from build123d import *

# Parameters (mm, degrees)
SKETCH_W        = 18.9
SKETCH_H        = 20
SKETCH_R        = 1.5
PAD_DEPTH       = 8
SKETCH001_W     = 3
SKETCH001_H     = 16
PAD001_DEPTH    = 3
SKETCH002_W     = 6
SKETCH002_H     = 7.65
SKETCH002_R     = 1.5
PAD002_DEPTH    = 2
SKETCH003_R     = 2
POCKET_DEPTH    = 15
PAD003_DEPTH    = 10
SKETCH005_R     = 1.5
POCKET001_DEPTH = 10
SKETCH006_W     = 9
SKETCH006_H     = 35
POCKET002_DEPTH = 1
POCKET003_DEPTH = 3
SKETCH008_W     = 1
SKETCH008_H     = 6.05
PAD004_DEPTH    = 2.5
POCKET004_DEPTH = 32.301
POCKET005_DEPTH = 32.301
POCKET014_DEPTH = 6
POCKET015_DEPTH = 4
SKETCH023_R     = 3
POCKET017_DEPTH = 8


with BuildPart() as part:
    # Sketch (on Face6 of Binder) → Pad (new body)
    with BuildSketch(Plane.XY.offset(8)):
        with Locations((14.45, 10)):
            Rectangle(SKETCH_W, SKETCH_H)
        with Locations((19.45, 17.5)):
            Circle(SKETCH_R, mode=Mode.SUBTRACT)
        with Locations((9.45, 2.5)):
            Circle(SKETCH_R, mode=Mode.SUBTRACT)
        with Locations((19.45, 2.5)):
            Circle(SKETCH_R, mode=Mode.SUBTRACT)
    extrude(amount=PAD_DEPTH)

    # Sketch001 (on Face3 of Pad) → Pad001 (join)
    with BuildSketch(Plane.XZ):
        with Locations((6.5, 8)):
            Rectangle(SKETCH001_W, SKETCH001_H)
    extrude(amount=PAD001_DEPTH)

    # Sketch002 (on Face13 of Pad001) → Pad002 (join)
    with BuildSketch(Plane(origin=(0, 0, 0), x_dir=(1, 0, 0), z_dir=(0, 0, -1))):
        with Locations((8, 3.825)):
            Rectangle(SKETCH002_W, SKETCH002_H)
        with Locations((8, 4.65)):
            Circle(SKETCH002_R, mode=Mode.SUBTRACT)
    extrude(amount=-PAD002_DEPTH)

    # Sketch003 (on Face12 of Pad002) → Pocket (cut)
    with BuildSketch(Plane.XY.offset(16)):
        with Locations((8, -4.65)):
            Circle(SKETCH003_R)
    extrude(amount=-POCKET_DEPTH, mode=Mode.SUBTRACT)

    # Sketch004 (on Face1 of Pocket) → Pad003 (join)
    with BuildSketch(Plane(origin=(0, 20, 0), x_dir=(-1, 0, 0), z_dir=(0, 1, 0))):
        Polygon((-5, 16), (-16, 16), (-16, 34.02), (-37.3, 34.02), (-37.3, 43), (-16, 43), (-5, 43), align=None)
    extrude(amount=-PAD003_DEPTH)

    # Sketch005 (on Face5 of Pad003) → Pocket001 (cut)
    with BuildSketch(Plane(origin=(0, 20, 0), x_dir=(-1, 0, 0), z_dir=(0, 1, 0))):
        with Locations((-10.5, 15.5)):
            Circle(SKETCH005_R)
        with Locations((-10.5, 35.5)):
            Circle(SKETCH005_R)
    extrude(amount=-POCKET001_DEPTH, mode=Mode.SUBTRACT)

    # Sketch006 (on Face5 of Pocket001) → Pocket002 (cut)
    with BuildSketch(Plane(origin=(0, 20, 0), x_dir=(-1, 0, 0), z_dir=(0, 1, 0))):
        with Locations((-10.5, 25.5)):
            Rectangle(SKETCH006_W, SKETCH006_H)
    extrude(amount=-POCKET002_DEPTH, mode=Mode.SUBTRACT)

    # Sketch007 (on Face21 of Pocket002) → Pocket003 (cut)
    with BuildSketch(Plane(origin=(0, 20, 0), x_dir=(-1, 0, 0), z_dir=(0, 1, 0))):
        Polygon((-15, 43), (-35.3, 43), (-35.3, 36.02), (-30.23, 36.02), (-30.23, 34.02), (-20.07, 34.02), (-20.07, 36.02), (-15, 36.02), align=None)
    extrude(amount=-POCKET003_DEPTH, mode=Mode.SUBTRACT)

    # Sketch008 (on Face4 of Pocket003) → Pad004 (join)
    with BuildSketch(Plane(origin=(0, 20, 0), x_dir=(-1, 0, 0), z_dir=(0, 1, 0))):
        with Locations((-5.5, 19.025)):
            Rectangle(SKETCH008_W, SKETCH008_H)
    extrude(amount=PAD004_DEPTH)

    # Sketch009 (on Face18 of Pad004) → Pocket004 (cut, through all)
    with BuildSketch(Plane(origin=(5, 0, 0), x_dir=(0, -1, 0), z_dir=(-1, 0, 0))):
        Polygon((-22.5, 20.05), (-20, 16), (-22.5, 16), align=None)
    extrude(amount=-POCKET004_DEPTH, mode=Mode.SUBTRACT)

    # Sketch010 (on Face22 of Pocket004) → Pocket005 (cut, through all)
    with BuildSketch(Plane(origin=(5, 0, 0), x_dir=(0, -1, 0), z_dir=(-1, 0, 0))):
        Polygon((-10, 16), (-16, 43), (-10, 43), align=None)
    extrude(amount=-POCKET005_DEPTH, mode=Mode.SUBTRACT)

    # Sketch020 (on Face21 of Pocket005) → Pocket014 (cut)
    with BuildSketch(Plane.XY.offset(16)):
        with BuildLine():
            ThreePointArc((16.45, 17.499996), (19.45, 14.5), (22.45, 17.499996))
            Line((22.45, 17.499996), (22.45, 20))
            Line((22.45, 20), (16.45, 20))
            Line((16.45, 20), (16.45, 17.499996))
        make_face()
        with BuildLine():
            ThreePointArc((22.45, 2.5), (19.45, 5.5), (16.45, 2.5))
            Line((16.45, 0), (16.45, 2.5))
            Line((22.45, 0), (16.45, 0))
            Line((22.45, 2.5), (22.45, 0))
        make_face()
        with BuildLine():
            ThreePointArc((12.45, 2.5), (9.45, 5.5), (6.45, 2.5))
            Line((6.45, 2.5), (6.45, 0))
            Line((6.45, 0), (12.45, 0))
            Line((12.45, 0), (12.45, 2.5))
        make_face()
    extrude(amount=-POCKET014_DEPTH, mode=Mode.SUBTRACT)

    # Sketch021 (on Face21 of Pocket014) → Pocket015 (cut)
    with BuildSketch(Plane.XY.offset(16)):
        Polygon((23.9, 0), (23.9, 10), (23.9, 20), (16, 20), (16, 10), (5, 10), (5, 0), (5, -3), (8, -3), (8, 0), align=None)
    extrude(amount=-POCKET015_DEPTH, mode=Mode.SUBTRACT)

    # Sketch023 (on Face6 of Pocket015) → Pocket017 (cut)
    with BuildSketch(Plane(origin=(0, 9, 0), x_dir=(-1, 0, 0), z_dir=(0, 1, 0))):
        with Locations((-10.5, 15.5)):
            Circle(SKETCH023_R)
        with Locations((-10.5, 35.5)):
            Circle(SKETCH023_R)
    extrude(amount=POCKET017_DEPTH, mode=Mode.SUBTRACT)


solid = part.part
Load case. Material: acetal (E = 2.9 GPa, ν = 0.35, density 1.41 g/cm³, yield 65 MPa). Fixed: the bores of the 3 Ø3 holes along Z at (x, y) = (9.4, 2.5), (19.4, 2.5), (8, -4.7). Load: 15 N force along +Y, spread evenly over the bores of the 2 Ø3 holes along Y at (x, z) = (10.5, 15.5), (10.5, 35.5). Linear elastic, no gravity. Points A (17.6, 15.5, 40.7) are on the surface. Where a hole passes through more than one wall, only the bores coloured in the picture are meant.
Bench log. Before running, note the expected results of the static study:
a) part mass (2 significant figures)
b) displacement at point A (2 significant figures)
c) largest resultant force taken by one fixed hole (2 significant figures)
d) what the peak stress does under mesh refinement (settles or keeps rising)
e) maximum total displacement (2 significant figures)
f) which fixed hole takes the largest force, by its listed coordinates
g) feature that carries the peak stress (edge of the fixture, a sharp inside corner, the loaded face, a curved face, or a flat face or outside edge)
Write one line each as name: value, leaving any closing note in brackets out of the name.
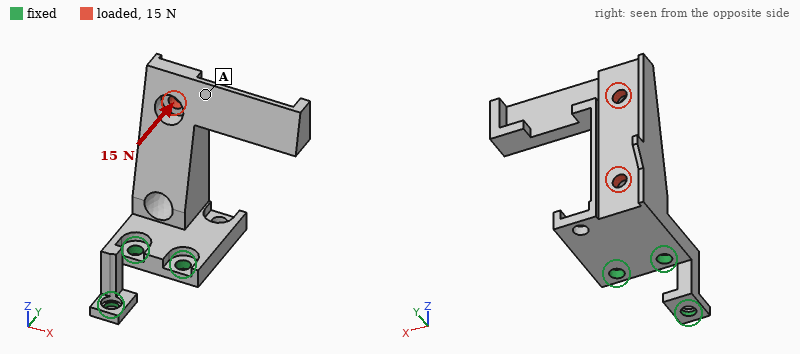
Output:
part mass: 5.4 g
displacement at point A: 0.51 mm
largest resultant force taken by one fixed hole: 13 N
what the peak stress does under mesh refinement: keeps rising
maximum total displacement: 0.57 mm
which fixed hole takes the largest force, by its listed coordinates: (9.4, 2.5)
feature that carries the peak stress: edge of the fixture
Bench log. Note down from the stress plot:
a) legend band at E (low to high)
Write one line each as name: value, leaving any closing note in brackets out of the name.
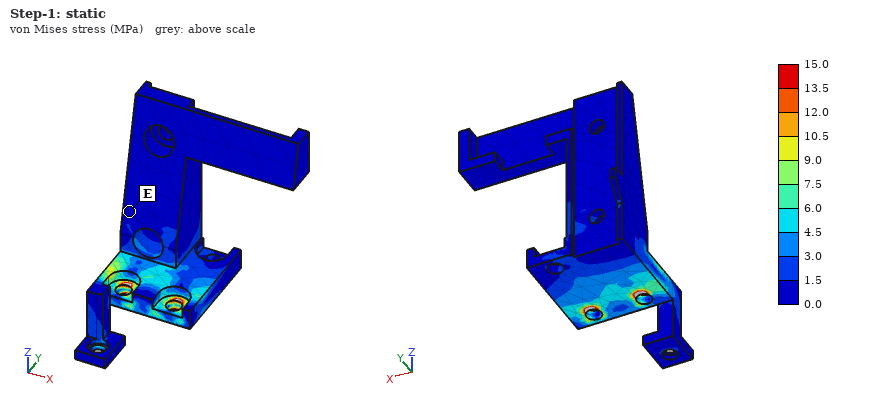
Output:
legend band at E: 0.0 to 1.5 MPa
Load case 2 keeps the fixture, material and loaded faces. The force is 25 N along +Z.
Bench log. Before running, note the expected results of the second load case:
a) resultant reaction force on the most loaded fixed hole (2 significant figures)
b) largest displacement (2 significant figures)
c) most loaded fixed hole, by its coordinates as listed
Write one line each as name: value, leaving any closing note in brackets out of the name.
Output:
resultant reaction force on the most loaded fixed hole: 30 N
largest displacement: 0.67 mm
most loaded fixed hole, by its coordinates as listed: (9.4, 2.5)
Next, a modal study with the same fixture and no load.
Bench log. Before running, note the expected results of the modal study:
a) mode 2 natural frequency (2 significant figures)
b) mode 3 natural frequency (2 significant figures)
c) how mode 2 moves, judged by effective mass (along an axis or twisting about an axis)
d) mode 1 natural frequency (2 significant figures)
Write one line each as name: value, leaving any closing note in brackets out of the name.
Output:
mode 2 natural frequency: 780 Hz
mode 3 natural frequency: 950 Hz
how mode 2 moves, judged by effective mass: along X
mode 1 natural frequency: 450 Hz
